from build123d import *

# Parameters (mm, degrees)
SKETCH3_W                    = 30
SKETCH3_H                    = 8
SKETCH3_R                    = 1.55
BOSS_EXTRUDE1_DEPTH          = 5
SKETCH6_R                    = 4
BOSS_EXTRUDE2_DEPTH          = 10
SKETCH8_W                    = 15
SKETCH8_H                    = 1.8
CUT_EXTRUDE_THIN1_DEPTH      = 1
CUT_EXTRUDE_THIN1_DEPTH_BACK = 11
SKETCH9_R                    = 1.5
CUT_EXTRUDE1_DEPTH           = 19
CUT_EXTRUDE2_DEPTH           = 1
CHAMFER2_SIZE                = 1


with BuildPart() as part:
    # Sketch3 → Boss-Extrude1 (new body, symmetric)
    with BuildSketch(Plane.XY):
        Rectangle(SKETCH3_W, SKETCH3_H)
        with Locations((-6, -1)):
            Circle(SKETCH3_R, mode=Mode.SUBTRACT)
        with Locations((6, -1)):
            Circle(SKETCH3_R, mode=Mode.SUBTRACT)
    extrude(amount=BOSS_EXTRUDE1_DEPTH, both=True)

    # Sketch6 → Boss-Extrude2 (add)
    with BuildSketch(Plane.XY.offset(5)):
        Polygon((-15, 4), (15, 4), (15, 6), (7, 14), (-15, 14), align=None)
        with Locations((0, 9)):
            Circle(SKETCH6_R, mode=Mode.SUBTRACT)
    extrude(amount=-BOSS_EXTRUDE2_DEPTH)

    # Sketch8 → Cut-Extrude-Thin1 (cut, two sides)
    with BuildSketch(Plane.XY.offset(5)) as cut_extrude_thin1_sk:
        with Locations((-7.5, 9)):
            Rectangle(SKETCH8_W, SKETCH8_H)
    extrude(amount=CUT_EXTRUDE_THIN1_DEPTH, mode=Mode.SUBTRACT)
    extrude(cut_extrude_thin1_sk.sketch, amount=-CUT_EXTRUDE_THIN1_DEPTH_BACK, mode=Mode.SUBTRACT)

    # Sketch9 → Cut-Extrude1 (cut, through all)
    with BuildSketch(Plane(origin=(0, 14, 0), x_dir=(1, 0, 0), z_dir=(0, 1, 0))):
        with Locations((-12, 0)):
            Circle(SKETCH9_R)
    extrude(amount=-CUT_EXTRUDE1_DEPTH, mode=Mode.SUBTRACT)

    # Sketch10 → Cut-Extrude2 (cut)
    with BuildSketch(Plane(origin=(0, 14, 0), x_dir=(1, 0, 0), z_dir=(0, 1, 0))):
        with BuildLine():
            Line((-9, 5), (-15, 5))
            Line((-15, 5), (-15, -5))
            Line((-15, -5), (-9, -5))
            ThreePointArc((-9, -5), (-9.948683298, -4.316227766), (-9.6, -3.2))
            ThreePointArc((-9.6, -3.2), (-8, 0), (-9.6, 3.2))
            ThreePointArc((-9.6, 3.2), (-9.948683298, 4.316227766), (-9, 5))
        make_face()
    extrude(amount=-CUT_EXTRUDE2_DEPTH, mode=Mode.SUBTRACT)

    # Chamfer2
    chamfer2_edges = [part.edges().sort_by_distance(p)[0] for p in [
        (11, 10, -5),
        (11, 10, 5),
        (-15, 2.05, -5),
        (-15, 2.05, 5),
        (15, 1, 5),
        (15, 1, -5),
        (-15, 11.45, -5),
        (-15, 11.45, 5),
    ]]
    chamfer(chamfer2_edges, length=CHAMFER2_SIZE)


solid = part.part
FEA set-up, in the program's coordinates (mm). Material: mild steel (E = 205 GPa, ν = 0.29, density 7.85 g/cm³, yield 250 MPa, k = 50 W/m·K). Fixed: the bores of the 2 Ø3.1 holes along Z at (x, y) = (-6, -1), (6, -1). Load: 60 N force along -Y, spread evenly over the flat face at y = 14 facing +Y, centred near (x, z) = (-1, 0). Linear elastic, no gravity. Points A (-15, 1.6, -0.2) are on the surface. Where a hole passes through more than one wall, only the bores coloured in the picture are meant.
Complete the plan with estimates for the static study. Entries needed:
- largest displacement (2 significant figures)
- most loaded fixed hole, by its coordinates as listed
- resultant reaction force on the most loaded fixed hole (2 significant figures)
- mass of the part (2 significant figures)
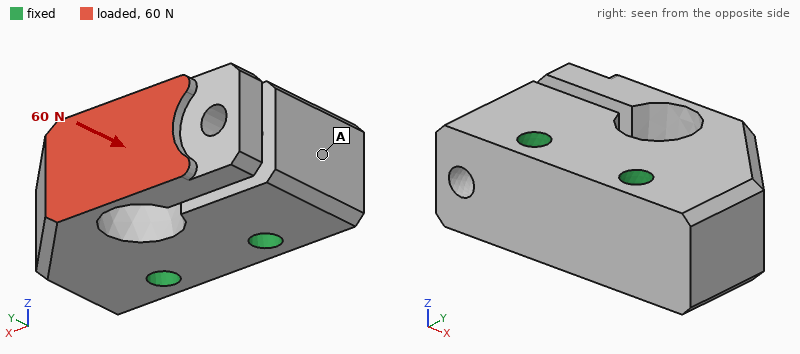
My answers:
50 µm
(6, -1)
42 N
32 g
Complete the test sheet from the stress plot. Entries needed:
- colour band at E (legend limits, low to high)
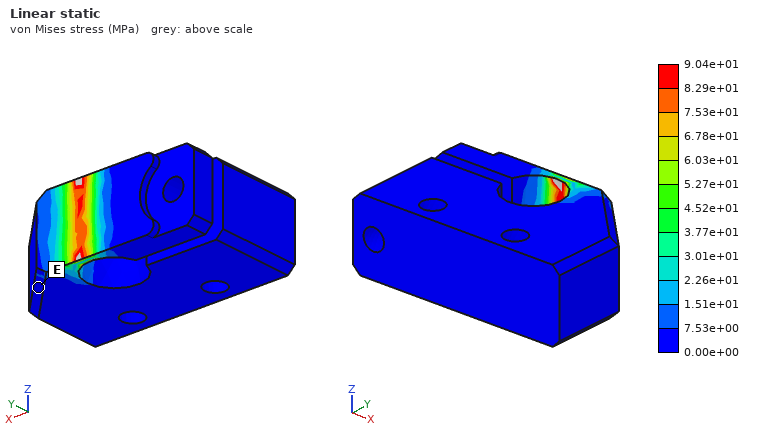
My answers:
0.00e+00 to 7.53e+00 MPa
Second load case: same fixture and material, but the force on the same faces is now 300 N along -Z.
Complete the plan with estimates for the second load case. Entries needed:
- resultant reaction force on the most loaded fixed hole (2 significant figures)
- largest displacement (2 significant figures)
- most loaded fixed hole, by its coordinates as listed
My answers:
200 N
19 µm
(6, -1)
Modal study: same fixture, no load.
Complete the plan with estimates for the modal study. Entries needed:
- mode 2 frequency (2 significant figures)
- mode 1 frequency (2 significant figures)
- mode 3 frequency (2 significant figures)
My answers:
7700 Hz
2200 Hz
13 kHz
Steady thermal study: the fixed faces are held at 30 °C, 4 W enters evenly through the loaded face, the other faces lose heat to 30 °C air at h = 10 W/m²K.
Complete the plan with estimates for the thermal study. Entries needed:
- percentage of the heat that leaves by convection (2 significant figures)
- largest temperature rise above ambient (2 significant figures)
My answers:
4.6 %
41 K
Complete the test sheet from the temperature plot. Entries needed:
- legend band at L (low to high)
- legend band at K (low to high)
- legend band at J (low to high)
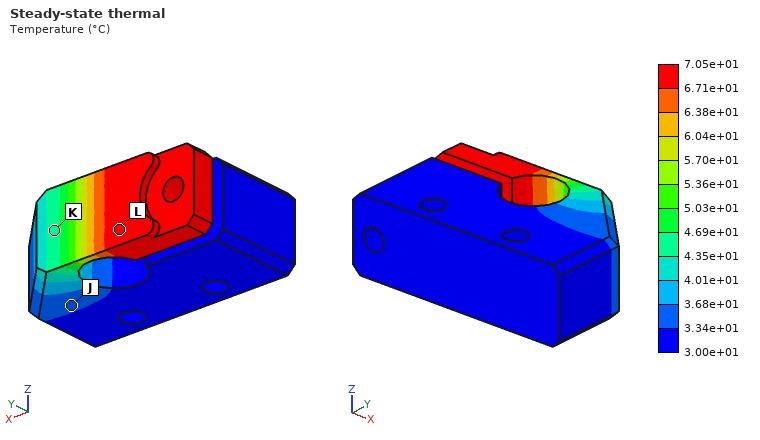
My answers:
6.71e+01 to 7.05e+01 °C
4.35e+01 to 4.69e+01 °C
3.34e+01 to 3.68e+01 °C
